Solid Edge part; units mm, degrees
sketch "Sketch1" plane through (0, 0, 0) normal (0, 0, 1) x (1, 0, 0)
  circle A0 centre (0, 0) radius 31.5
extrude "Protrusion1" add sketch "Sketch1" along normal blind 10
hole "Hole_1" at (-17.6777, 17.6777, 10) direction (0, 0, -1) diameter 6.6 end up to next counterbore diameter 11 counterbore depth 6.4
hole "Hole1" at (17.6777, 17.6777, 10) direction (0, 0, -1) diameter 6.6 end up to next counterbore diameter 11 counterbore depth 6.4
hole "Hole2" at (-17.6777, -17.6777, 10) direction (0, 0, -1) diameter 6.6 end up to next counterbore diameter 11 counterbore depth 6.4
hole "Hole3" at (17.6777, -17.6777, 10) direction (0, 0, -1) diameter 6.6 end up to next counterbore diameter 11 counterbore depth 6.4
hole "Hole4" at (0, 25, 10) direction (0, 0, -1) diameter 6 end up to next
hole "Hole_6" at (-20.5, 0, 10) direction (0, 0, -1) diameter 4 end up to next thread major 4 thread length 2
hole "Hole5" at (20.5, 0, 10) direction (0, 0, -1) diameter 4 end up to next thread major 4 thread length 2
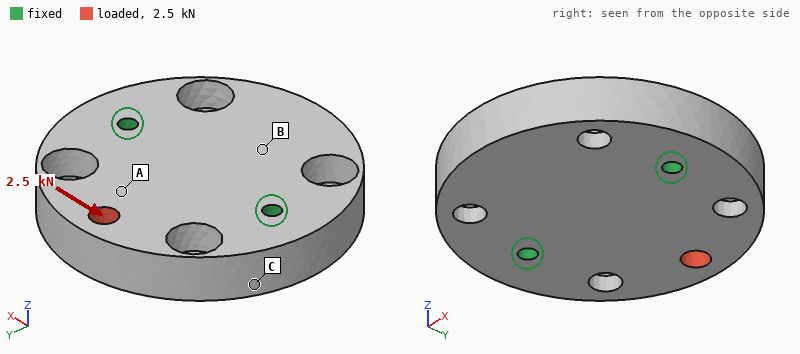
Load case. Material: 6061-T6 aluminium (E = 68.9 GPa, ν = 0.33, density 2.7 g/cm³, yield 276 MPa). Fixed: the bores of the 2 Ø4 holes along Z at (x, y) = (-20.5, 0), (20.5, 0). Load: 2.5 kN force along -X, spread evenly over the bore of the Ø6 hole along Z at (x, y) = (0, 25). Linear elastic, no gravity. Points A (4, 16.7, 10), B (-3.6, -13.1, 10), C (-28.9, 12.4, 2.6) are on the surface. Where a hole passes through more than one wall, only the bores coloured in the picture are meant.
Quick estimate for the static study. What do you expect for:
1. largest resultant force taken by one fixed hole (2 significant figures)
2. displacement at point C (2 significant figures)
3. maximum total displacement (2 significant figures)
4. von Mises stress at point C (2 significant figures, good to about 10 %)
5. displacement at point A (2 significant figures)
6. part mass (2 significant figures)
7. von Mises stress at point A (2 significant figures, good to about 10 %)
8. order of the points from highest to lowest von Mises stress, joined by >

1.9 kN
4.2 µm
11 µm
8.1 MPa
5.4 µm
75 g
15 MPa
A > C > B
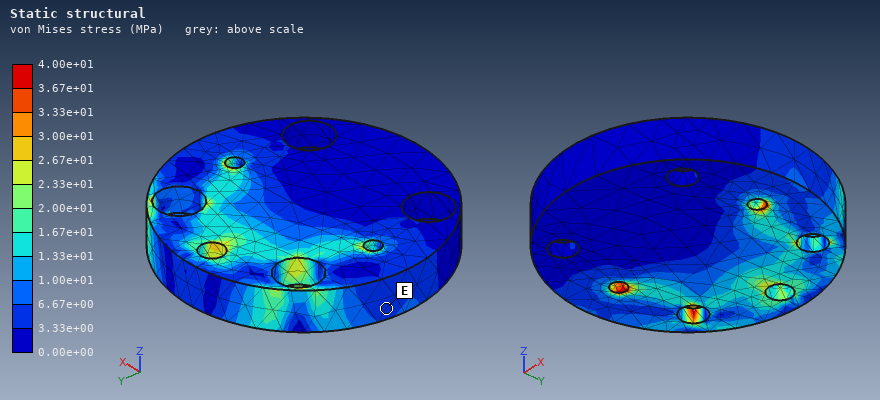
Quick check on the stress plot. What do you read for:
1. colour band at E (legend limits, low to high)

3.33e+00 to 6.67e+00 MPa
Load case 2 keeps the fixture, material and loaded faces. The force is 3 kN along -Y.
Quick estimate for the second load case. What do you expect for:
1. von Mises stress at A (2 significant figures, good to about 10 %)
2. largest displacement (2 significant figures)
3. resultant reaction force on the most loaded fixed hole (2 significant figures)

14 MPa
9.4 µm
1.5 kN
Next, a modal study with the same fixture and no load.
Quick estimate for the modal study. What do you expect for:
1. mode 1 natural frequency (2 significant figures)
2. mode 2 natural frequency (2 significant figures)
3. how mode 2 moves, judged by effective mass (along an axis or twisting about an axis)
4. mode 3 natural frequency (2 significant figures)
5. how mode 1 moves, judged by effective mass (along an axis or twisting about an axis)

6600 Hz
9100 Hz
along Z
17 kHz
twisting about X
